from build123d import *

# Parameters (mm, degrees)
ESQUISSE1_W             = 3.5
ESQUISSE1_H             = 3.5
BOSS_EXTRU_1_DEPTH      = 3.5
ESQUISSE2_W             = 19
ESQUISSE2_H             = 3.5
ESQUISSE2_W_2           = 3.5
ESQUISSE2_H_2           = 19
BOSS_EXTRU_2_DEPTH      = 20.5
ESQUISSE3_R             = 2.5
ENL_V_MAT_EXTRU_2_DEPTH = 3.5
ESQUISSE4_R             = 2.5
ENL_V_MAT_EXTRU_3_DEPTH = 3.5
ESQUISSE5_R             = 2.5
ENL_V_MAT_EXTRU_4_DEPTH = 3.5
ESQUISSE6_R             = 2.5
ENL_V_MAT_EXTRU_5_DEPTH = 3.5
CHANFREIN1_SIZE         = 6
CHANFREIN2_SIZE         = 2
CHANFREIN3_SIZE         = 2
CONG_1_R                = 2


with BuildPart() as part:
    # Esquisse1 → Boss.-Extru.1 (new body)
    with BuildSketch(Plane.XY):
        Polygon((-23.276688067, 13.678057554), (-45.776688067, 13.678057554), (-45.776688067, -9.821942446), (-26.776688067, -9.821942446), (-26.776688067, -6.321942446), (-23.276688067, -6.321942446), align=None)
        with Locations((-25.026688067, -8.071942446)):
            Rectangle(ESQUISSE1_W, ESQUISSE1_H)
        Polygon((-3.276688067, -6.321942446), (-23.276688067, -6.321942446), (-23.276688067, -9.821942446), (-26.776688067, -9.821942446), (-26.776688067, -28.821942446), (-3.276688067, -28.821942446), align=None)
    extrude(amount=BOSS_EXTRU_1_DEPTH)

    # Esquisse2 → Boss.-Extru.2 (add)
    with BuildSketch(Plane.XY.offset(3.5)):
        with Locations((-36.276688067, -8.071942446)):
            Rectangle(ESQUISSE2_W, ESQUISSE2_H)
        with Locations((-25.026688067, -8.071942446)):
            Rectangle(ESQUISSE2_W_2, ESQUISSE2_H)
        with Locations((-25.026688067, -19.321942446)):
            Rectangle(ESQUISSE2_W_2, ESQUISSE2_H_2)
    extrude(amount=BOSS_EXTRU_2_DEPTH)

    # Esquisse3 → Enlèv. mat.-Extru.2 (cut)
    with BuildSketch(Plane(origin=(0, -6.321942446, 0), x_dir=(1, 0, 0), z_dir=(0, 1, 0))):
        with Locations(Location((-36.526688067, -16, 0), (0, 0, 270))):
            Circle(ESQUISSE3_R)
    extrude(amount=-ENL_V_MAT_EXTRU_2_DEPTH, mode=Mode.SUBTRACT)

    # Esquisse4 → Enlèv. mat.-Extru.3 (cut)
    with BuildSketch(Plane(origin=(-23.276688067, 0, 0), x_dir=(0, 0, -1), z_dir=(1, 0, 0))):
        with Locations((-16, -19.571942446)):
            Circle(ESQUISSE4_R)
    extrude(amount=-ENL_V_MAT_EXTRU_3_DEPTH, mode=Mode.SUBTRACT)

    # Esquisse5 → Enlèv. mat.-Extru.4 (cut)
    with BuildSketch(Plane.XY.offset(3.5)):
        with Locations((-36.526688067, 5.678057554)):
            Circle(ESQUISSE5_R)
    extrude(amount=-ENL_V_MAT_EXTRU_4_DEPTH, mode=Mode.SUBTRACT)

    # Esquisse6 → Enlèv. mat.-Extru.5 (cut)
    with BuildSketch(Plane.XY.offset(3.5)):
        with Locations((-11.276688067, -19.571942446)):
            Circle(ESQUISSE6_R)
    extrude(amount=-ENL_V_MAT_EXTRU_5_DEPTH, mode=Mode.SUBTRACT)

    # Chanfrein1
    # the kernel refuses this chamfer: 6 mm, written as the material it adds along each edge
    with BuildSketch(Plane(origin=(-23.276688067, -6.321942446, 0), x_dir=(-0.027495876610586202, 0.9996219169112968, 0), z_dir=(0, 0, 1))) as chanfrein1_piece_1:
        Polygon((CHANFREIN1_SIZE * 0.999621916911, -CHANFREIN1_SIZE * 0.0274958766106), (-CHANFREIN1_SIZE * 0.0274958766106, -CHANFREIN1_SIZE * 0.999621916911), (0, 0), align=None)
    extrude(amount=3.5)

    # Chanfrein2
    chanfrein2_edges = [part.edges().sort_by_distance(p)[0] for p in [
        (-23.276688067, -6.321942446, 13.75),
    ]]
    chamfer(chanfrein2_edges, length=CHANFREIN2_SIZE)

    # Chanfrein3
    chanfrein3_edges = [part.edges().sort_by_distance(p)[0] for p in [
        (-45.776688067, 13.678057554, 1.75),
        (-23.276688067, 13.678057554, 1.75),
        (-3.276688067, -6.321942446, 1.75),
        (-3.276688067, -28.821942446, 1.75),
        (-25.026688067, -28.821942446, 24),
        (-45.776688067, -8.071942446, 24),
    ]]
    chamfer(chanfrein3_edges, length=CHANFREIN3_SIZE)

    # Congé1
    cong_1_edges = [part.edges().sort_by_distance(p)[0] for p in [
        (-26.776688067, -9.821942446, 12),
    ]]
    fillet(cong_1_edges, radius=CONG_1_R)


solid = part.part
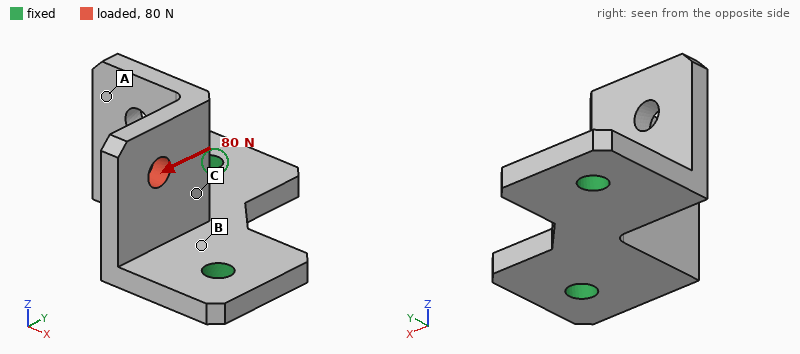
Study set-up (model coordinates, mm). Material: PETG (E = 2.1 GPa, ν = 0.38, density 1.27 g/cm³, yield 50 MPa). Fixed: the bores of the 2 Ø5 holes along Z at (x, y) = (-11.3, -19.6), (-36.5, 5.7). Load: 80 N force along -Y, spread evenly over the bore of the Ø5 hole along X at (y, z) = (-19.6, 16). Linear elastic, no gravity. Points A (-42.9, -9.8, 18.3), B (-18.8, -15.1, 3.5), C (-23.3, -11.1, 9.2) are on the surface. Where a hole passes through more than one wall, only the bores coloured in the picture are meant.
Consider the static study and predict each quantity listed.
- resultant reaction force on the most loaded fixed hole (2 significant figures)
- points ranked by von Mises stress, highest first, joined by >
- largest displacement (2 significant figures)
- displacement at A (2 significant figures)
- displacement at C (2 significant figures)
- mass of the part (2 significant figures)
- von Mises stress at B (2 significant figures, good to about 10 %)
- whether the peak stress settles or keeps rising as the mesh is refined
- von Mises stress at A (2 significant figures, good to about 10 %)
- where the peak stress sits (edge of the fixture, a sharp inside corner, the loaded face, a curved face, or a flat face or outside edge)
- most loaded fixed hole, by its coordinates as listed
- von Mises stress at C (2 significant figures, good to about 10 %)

54 N
B > C > A
0.64 mm
0.30 mm
0.19 mm
8.1 g
7.4 MPa
keeps rising
1.3 MPa
edge of the fixture
(-36.5, 5.7)
4.6 MPa
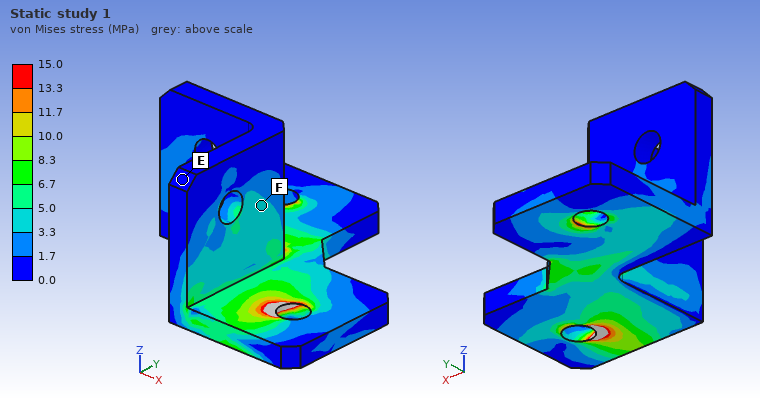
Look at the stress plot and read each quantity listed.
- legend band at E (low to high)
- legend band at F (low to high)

0.0 to 1.7 MPa
3.3 to 5.0 MPa
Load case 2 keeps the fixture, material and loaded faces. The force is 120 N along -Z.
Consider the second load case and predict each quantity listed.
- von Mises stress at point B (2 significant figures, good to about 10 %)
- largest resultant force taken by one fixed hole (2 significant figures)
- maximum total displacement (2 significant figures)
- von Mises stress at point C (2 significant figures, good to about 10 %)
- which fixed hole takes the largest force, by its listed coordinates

7.2 MPa
97 N
0.64 mm
3.5 MPa
(-11.3, -19.6)
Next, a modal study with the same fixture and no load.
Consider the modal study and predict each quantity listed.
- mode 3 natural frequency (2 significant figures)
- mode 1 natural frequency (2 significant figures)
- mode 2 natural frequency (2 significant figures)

2100 Hz
1100 Hz
2000 Hz
